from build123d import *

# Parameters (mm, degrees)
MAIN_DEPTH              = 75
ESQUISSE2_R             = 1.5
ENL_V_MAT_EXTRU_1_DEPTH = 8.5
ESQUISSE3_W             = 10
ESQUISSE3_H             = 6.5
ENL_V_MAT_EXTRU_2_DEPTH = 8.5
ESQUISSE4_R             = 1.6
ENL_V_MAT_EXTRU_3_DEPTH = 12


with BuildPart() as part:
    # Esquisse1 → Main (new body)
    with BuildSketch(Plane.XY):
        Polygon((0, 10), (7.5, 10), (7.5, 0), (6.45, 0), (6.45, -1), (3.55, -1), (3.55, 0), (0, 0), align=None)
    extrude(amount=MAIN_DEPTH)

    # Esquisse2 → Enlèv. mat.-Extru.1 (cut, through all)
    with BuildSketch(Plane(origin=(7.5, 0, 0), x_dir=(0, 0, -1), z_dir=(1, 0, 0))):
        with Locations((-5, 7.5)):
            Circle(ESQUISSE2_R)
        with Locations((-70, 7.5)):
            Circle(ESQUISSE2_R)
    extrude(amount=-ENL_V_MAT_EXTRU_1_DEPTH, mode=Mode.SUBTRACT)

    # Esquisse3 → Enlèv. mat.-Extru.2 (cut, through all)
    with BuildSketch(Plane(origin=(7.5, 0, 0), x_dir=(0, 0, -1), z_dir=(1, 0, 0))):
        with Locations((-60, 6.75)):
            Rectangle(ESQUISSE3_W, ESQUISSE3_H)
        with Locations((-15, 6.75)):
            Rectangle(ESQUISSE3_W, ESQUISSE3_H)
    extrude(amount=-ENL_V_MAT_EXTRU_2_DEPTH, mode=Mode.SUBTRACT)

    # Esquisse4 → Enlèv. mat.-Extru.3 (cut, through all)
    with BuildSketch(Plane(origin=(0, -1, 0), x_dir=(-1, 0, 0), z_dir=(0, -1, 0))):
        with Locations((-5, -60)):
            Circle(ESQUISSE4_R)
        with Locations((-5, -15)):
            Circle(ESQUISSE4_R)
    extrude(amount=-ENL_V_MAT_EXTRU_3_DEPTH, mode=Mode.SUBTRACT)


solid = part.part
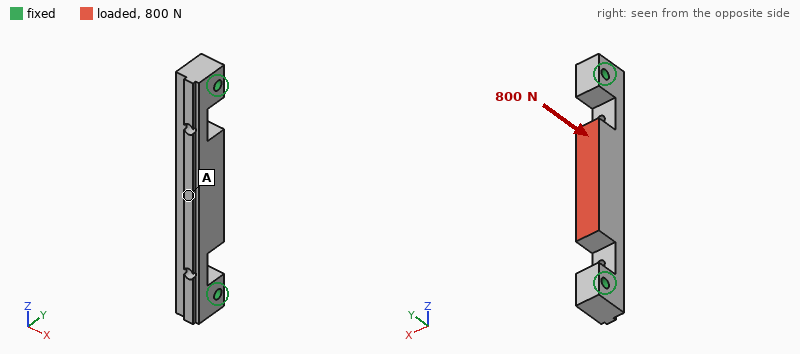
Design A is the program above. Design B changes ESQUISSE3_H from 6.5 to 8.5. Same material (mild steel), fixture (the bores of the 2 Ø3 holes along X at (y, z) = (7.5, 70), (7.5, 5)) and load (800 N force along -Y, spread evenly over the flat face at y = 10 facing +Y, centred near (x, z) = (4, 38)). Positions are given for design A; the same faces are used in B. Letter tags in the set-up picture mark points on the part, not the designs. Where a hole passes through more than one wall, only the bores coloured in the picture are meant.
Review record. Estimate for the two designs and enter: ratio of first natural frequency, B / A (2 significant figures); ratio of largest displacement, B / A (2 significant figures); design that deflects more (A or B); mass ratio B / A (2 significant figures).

0.75
1.6
B
0.97
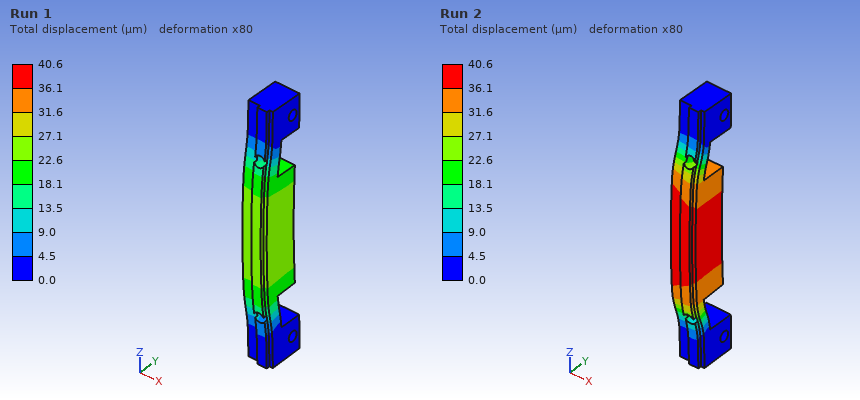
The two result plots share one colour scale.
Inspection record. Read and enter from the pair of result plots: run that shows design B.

Run 2
